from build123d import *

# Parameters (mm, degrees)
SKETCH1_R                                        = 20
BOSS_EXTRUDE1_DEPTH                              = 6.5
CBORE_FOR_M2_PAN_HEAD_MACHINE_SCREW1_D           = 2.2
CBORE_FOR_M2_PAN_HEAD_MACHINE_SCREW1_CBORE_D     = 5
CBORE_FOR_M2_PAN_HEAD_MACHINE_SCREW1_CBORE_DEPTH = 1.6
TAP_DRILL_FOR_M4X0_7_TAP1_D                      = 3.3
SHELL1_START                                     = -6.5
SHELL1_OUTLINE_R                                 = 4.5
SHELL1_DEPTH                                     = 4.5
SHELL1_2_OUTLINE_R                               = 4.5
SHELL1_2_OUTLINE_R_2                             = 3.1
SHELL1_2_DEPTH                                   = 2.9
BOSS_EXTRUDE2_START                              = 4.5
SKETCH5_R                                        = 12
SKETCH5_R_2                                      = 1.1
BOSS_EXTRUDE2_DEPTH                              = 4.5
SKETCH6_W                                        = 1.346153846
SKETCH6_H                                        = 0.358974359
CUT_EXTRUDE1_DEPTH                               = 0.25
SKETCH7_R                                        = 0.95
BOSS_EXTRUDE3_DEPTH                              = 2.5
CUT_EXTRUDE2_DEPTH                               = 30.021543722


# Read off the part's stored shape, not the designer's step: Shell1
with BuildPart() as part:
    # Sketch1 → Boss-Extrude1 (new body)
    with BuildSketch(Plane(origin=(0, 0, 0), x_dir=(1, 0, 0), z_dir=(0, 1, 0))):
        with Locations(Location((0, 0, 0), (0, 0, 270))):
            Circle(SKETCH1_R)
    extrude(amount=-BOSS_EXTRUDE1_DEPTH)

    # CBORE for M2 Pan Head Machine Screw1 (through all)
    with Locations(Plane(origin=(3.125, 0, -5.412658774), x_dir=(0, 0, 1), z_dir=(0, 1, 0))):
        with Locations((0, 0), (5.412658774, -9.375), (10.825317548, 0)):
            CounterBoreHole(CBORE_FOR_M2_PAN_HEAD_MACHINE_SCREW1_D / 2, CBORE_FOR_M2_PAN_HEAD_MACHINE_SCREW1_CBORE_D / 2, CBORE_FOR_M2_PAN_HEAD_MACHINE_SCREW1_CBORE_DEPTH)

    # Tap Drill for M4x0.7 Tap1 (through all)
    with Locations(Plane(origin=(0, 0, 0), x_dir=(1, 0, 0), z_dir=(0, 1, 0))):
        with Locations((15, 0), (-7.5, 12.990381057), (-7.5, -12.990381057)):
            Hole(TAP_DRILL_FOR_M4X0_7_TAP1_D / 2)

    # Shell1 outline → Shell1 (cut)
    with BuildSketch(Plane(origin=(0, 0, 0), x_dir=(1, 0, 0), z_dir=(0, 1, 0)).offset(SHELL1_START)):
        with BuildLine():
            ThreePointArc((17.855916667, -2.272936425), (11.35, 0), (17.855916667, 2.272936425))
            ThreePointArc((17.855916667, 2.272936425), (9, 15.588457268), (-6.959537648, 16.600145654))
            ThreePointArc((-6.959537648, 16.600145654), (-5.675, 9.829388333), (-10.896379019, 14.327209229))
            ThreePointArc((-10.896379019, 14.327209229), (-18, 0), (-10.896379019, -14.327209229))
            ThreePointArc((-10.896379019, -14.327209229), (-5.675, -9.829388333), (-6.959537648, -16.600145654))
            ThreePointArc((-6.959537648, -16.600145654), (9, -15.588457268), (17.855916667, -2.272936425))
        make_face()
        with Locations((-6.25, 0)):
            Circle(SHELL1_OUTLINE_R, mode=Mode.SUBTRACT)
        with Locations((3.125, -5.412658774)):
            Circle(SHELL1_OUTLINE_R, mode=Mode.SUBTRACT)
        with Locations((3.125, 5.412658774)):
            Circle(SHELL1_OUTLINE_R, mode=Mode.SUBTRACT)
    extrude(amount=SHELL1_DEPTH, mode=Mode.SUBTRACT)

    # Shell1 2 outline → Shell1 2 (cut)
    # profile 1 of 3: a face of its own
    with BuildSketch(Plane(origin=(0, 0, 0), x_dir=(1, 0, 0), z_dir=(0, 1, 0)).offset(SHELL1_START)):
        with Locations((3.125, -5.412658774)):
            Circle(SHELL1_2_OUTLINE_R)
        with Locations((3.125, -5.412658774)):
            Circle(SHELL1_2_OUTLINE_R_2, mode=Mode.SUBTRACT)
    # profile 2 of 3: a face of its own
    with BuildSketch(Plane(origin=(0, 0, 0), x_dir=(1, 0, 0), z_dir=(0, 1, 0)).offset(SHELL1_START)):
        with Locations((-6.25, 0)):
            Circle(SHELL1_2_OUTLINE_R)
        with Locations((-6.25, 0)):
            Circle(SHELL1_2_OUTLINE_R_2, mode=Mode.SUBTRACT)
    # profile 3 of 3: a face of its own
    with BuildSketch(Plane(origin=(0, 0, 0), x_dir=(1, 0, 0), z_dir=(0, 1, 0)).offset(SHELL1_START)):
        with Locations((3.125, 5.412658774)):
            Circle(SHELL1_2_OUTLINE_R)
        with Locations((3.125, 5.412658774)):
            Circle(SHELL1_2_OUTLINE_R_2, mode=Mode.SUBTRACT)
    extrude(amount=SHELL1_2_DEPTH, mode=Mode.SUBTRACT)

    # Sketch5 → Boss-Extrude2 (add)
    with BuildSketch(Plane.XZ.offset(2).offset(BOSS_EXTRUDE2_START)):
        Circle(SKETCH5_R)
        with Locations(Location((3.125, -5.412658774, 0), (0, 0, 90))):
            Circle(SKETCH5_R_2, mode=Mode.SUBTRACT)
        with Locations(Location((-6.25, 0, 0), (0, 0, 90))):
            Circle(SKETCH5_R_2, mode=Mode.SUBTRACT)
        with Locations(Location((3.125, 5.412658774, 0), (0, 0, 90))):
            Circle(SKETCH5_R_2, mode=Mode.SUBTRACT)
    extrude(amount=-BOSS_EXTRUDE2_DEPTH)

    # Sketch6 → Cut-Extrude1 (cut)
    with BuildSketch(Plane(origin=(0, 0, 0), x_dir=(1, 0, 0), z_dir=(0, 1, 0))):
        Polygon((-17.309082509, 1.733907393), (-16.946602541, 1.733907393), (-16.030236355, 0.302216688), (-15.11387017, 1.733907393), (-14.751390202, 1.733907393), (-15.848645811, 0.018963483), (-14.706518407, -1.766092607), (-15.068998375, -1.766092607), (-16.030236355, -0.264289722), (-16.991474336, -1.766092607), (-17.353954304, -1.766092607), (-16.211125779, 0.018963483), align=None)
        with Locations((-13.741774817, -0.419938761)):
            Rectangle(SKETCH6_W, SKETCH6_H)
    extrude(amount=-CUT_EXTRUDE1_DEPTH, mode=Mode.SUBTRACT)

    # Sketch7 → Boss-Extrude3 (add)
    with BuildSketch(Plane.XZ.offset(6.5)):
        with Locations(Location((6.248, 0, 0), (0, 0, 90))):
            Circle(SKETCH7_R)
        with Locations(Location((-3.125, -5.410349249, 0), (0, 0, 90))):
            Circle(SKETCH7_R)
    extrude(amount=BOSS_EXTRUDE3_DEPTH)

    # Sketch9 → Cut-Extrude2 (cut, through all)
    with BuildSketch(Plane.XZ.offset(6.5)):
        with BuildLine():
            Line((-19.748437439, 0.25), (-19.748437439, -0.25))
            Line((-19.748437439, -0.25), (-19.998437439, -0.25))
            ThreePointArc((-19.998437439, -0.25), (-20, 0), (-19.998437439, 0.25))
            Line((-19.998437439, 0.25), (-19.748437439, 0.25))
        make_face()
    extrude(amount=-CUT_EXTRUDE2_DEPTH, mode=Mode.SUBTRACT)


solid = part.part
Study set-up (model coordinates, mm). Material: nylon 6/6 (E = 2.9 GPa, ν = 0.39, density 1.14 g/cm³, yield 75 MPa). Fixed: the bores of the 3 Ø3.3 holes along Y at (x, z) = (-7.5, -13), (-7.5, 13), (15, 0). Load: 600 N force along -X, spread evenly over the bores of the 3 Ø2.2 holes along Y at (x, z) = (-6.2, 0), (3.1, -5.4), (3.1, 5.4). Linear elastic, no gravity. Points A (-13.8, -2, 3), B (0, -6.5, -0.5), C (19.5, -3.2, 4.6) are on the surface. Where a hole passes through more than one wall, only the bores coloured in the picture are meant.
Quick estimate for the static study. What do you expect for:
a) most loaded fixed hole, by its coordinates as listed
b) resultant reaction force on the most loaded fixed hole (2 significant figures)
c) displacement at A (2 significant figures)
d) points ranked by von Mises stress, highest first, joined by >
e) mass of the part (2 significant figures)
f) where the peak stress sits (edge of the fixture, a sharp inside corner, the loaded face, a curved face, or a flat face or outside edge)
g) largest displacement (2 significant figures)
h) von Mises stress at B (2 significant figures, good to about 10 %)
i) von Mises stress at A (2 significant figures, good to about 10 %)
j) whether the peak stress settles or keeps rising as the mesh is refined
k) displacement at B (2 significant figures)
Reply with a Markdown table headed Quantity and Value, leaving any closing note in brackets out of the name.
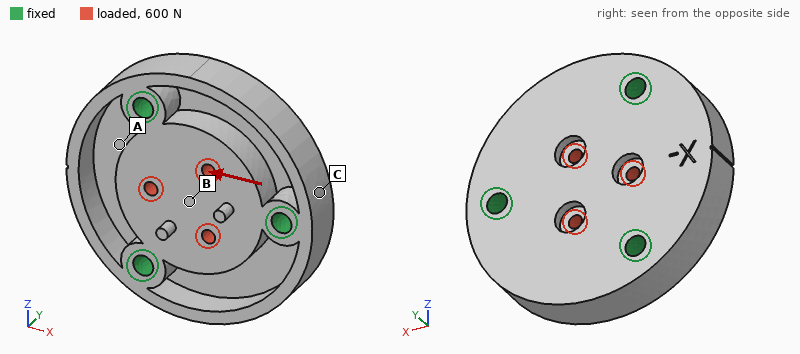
| Quantity | Value |
|---|---|
| most loaded fixed hole, by its coordinates as listed | (15, 0) |
| resultant reaction force on the most loaded fixed hole | 250 N |
| displacement at A | 19 µm |
| points ranked by von Mises stress, highest first, joined by > | B > A > C |
| mass of the part | 6.7 g |
| where the peak stress sits | edge of the fixture |
| largest displacement | 34 µm |
| von Mises stress at B | 4.8 MPa |
| von Mises stress at A | 3.0 MPa |
| whether the peak stress settles or keeps rising as the mesh is refined | keeps rising |
| displacement at B | 22 µm |
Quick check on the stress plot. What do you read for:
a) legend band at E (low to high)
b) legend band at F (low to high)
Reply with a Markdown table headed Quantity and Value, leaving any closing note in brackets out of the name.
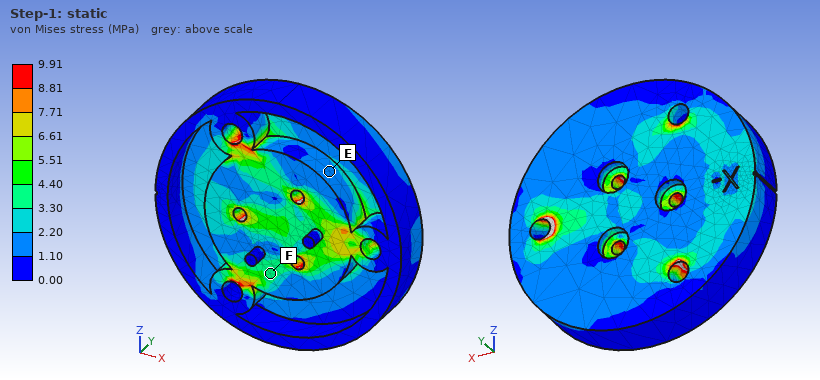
| Quantity | Value |
|---|---|
| legend band at E | 1.10 to 2.20 MPa |
| legend band at F | 3.30 to 4.40 MPa |
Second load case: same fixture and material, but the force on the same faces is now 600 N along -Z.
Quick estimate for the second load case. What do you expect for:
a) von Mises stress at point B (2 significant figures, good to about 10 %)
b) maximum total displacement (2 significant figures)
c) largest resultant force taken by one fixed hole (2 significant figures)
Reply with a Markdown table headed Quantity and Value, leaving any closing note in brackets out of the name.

| Quantity | Value |
|---|---|
| von Mises stress at point B | 4.8 MPa |
| maximum total displacement | 31 µm |
| largest resultant force taken by one fixed hole | 230 N |
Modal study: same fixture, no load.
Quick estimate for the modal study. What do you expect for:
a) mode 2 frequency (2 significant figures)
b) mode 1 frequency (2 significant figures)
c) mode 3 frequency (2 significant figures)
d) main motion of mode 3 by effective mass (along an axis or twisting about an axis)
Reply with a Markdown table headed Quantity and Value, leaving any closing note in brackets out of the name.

| Quantity | Value |
|---|---|
| mode 2 frequency | 5900 Hz |
| mode 1 frequency | 5900 Hz |
| mode 3 frequency | 6600 Hz |
| main motion of mode 3 by effective mass | along Y |
